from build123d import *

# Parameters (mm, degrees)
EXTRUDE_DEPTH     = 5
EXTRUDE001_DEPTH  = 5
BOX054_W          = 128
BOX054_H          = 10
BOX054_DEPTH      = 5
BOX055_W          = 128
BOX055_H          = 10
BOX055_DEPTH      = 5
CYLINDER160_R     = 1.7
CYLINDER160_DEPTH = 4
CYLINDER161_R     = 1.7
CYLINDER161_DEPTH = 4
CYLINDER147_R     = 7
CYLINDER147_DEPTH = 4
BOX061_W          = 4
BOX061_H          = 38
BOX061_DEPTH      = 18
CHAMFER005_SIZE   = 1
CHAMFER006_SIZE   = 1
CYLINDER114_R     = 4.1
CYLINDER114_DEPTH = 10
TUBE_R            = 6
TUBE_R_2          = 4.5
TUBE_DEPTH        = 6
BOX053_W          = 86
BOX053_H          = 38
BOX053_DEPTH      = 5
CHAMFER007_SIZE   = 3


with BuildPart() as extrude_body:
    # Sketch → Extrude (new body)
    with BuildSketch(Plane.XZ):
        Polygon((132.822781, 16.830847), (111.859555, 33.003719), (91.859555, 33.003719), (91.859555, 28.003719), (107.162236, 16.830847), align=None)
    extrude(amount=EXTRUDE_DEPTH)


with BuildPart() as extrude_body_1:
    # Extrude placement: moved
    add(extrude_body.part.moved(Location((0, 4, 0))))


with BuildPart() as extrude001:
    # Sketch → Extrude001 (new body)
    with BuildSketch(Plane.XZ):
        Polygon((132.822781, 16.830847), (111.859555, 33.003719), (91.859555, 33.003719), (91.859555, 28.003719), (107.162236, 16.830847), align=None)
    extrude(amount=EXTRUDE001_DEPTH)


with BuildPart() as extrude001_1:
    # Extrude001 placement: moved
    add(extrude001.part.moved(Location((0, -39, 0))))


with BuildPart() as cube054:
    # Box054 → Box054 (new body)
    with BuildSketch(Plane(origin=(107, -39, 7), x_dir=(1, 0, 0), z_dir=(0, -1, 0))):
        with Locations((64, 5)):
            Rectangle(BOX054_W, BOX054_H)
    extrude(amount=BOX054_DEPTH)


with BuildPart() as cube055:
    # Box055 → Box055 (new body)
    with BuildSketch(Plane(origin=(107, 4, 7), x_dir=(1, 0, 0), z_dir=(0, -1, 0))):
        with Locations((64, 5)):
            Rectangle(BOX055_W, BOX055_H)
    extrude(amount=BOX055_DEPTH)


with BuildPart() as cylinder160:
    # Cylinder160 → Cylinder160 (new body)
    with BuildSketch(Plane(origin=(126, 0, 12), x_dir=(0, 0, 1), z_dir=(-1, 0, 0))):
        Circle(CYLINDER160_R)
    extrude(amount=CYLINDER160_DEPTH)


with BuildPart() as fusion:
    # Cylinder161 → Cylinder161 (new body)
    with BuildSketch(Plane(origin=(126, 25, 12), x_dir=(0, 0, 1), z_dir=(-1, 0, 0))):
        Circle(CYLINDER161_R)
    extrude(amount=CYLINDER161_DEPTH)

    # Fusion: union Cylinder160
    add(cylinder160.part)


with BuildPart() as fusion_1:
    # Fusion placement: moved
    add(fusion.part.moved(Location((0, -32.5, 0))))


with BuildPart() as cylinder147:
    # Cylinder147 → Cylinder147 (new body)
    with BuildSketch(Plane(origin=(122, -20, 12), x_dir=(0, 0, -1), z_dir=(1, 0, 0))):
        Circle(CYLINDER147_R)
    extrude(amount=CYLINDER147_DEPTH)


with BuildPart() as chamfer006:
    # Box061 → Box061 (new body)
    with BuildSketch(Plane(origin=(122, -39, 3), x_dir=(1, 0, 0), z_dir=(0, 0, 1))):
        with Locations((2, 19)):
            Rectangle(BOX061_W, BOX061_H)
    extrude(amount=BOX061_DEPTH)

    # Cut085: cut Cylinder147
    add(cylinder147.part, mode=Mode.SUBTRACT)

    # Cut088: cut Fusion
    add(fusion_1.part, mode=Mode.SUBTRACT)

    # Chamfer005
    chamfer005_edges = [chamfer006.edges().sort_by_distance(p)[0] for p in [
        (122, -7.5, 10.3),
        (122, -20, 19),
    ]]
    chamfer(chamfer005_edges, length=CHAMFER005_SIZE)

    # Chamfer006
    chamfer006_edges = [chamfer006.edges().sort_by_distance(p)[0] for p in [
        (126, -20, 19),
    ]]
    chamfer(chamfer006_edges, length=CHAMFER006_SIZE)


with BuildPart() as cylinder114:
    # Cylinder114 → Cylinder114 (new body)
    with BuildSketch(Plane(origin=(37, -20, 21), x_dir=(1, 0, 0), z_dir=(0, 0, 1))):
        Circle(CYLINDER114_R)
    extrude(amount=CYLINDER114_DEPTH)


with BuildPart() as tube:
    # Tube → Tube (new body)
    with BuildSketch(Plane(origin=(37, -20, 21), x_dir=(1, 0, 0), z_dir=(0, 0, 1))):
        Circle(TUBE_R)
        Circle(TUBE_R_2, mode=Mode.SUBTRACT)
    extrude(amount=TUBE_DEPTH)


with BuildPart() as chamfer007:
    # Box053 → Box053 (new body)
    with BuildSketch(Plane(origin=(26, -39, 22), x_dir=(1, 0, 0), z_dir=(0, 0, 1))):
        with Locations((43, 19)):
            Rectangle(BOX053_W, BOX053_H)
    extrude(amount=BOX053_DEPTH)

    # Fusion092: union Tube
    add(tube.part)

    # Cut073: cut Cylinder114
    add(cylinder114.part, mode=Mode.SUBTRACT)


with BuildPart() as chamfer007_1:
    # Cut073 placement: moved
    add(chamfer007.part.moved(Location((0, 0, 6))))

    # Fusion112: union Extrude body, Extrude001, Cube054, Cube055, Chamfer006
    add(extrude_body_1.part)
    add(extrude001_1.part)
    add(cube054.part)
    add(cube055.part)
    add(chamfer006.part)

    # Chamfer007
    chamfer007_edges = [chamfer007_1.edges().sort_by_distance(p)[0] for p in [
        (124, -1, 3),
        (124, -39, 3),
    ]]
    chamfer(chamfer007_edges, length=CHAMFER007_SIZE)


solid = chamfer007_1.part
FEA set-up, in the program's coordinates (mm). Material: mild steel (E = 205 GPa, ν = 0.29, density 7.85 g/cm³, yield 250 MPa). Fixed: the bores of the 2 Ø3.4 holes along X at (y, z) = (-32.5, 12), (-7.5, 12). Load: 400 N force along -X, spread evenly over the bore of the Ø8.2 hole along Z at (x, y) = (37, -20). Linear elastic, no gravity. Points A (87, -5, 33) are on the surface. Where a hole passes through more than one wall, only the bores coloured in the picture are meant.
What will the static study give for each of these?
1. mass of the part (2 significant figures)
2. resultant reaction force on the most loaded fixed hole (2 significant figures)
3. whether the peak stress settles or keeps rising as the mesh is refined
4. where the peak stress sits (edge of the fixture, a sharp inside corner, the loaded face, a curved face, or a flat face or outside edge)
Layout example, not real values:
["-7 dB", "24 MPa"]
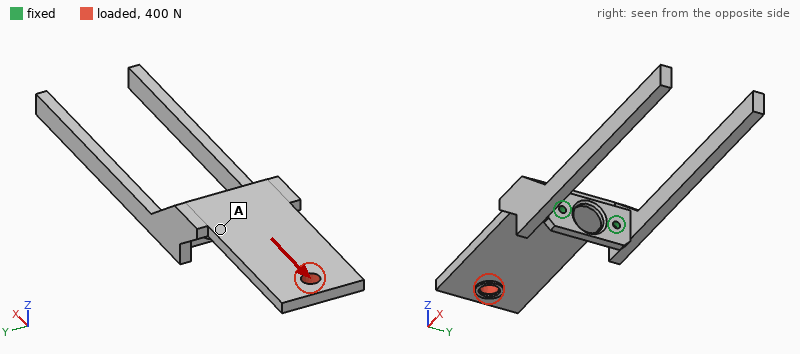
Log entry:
["270 g", "200 N", "keeps rising", "edge of the fixture"]
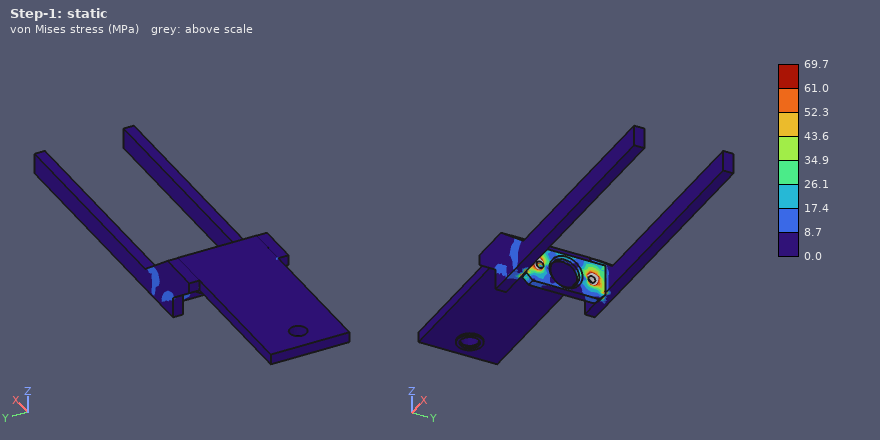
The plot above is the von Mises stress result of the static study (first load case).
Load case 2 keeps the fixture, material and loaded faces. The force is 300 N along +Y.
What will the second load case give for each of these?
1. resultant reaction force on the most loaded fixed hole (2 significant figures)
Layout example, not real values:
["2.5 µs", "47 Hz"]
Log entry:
["690 N"]
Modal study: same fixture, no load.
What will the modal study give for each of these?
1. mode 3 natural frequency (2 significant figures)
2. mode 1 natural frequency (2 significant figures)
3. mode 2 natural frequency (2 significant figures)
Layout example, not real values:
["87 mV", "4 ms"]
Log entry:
["380 Hz", "300 Hz", "320 Hz"]
